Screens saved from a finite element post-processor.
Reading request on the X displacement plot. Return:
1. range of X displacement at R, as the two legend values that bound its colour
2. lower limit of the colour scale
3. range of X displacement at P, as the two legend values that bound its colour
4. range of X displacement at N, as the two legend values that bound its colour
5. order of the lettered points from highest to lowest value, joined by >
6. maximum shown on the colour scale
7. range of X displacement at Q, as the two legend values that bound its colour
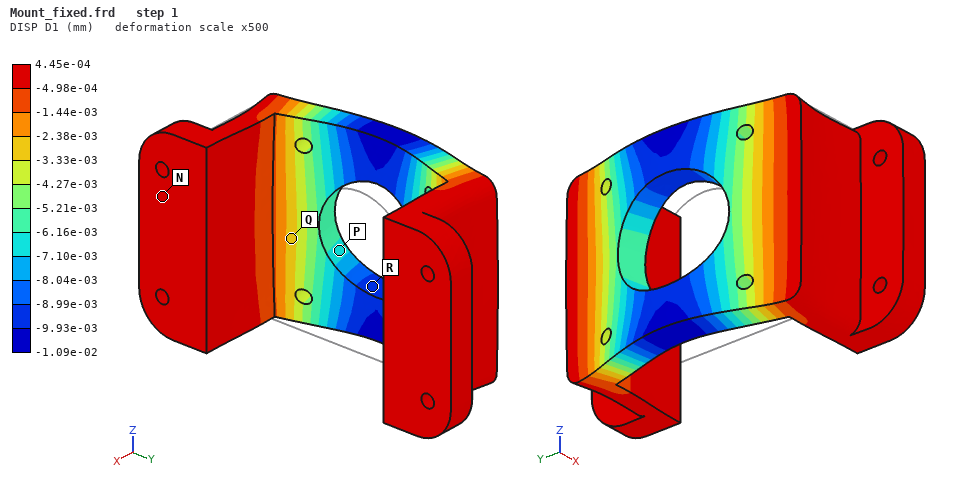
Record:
-9.93e-03 to -8.99e-03 mm
-1.09e-02 mm
-7.10e-03 to -6.16e-03 mm
-4.98e-04 to 4.45e-04 mm
N > Q > P > R
4.45e-04 mm
-3.33e-03 to -2.38e-03 mm
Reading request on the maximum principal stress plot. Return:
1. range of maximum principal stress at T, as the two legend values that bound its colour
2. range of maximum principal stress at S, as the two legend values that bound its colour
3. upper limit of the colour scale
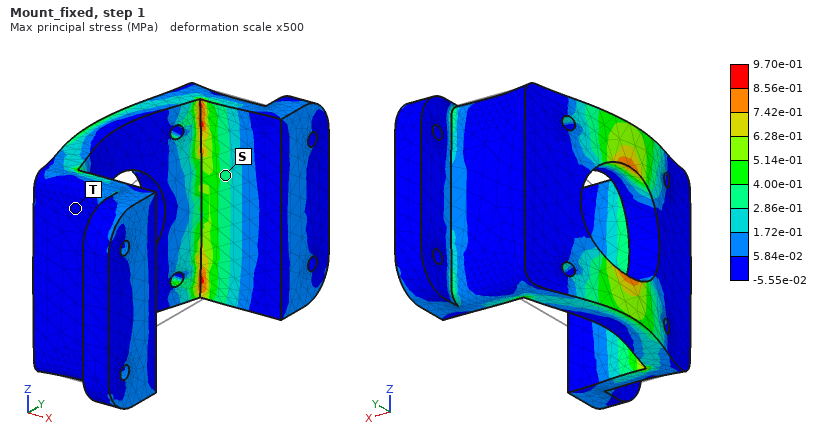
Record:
-5.55e-02 to 5.84e-02 MPa
2.86e-01 to 4.00e-01 MPa
9.70e-01 MPa
